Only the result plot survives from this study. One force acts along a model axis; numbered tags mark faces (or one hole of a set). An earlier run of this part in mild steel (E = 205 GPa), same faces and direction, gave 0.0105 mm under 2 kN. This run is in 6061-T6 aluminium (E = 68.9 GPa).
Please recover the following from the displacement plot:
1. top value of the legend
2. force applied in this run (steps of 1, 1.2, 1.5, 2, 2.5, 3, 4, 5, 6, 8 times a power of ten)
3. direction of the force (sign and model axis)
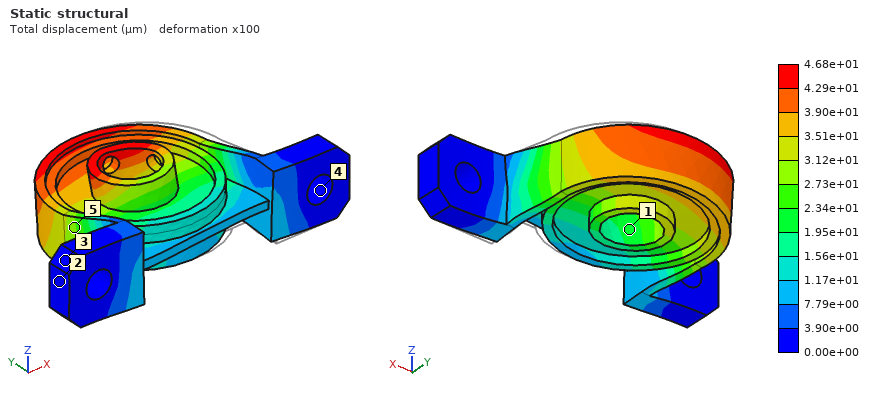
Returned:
4.68e+01 µm
3 kN
-X
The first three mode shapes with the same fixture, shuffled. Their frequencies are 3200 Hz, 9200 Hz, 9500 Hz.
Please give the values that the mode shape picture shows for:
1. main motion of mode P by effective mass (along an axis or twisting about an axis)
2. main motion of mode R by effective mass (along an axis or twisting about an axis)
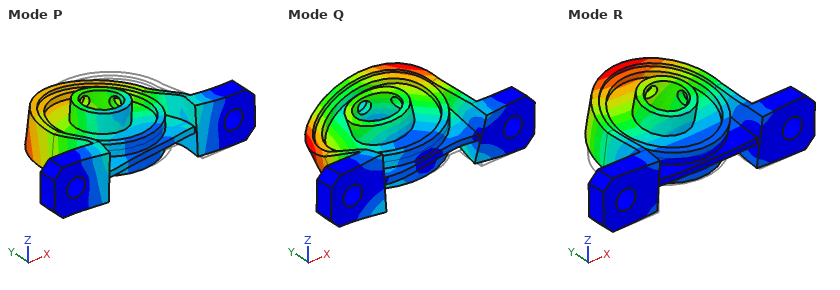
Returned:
along X
along Z
